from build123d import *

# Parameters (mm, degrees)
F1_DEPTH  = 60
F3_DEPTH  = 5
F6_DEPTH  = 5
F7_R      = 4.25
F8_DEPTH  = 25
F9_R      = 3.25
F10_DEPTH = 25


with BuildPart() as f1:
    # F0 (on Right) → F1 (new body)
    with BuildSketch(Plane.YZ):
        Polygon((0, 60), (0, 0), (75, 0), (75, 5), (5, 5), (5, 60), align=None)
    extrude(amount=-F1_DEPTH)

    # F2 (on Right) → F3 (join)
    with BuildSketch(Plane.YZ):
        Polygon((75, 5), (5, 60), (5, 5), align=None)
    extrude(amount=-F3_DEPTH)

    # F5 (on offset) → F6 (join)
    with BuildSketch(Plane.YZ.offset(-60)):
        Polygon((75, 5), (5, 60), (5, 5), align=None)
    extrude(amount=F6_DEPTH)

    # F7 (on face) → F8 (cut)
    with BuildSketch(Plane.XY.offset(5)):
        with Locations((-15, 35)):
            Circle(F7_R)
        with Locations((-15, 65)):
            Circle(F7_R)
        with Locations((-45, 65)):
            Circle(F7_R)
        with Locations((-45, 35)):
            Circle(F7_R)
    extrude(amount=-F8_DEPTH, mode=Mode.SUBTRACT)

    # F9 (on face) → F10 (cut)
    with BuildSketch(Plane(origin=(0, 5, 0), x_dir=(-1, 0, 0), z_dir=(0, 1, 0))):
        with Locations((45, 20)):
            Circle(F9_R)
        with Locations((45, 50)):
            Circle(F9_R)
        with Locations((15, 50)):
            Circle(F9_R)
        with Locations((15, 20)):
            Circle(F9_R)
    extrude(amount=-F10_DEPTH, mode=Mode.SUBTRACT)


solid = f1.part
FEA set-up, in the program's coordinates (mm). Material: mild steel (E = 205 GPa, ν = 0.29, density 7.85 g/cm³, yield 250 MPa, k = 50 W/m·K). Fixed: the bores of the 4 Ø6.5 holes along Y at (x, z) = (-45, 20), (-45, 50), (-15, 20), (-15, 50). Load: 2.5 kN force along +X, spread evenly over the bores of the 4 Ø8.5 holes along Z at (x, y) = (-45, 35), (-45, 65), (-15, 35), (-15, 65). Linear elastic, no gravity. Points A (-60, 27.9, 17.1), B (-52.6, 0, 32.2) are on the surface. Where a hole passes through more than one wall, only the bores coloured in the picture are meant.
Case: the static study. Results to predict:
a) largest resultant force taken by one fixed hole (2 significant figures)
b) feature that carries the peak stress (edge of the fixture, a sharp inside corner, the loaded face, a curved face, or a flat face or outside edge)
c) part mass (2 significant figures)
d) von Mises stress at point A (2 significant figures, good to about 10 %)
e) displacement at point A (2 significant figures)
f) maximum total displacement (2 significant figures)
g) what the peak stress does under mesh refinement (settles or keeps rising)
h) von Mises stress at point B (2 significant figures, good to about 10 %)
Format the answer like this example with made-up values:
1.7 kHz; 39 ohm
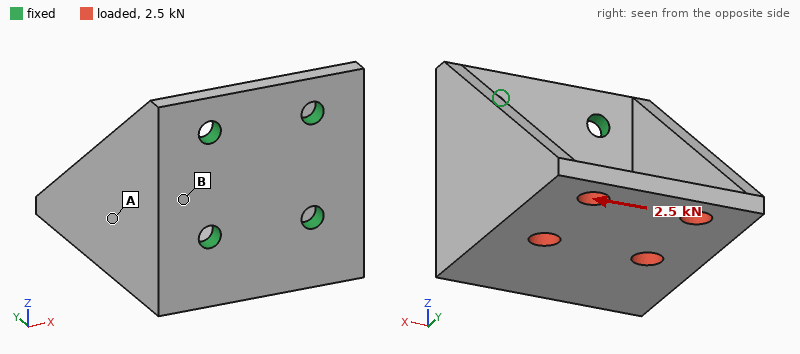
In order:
3.7 kN; edge of the fixture; 440 g; 22 MPa; 0.046 mm; 0.11 mm; keeps rising; 49 MPa
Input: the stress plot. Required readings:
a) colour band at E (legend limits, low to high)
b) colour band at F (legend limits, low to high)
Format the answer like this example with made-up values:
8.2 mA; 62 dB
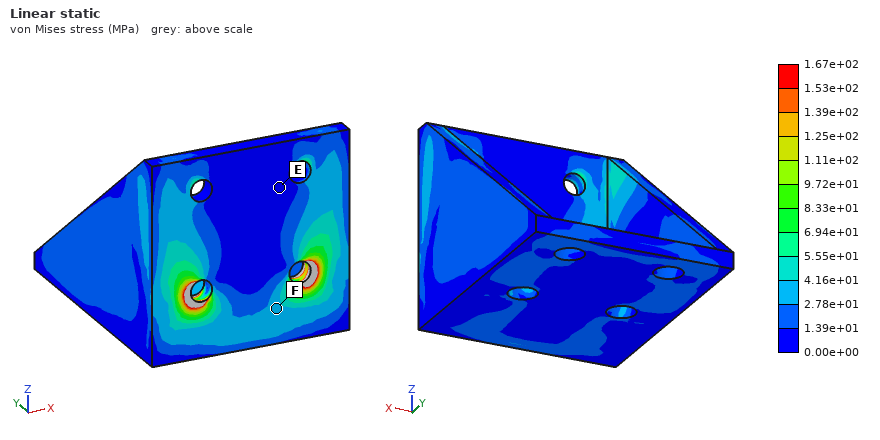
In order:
0.00e+00 to 1.39e+01 MPa; 2.78e+01 to 4.16e+01 MPa
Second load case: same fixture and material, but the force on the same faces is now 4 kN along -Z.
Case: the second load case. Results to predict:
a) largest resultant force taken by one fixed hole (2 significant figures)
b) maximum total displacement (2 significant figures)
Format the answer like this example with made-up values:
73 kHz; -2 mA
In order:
2.9 kN; 0.17 mm
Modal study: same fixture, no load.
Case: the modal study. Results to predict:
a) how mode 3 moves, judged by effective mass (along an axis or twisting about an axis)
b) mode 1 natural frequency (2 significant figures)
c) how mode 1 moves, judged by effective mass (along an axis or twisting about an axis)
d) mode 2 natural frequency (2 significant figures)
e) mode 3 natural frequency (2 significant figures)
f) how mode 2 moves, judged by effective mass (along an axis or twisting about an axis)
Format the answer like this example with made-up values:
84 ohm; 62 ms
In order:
along Y; 2000 Hz; along X; 2500 Hz; 4600 Hz; along Z
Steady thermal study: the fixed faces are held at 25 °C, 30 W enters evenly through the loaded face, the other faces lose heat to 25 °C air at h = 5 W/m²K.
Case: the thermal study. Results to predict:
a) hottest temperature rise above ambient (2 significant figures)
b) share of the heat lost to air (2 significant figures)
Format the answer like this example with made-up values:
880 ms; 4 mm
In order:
71 K; 11 %
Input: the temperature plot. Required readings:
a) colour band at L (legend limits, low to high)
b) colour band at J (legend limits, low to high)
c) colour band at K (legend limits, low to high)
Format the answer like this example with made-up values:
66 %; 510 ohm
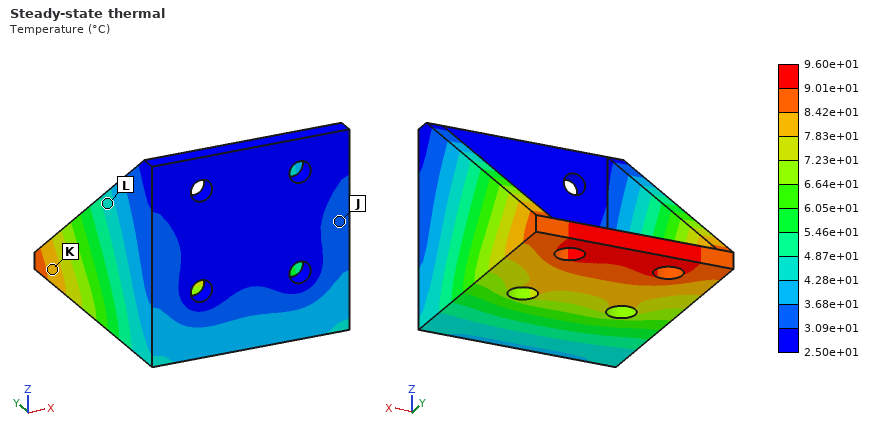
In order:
4.28e+01 to 4.87e+01 °C; 3.09e+01 to 3.68e+01 °C; 7.83e+01 to 8.42e+01 °C
